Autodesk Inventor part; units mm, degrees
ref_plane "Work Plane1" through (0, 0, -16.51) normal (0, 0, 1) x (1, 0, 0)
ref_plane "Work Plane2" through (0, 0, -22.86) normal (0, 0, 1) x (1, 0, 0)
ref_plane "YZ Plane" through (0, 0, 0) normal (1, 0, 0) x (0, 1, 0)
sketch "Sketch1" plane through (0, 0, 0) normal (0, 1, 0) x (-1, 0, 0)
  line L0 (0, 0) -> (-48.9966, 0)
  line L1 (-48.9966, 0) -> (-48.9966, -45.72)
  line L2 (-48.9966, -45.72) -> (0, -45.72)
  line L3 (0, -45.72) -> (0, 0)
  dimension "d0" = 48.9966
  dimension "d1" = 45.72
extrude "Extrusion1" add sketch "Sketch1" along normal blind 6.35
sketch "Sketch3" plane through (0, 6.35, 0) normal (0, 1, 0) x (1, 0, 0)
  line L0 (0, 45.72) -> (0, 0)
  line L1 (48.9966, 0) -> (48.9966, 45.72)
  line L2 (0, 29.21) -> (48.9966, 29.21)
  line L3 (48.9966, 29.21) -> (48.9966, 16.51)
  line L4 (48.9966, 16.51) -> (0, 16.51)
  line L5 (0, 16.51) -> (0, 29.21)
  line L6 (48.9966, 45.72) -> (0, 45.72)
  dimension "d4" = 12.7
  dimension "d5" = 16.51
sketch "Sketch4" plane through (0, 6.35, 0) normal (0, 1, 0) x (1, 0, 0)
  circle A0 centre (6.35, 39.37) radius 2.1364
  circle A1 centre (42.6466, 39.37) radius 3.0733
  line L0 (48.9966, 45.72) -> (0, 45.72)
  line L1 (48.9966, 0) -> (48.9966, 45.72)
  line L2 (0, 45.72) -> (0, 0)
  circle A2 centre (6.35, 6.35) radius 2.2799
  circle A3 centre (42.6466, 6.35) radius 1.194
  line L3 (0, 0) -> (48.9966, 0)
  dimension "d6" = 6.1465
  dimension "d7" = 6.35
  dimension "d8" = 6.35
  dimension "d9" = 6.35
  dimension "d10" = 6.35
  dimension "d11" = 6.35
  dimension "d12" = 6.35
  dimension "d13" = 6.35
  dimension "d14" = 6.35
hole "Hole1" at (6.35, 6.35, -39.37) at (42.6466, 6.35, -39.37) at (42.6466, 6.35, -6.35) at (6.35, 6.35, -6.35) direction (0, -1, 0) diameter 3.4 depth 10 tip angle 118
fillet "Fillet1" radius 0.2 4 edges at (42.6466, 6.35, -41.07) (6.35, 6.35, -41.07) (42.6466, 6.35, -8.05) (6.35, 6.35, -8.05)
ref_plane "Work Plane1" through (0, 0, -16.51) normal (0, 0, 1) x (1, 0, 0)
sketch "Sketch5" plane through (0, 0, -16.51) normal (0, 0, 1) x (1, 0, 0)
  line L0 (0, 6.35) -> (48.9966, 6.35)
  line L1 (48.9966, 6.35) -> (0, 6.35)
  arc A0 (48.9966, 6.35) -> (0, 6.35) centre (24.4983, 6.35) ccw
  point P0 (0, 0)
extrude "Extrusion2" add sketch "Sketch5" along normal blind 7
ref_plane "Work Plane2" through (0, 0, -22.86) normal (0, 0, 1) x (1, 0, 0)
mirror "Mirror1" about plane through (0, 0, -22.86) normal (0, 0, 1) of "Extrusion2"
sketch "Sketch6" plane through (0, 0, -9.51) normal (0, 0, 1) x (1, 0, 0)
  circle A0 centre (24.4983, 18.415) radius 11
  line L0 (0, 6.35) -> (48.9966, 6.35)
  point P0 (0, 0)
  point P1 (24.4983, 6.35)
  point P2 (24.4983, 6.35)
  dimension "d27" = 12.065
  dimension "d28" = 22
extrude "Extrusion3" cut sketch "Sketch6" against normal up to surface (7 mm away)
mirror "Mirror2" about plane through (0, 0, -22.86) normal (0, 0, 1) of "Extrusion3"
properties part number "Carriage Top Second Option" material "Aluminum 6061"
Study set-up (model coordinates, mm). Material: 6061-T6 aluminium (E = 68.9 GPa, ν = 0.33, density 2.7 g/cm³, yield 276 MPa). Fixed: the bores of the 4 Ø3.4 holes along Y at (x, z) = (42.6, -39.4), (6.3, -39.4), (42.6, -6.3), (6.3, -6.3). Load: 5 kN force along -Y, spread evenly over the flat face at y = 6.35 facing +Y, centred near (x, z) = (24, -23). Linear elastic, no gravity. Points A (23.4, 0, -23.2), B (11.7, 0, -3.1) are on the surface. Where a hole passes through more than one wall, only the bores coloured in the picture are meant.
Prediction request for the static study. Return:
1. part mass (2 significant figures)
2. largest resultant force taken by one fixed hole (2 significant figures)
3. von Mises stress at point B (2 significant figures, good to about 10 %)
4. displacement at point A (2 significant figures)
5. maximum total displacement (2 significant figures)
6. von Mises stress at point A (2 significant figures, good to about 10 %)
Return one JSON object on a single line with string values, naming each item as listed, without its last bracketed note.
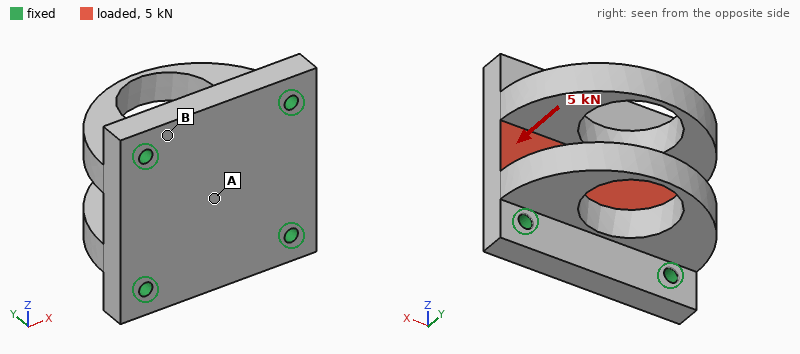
{"part mass": "59 g", "largest resultant force taken by one fixed hole": "1.3 kN", "von Mises stress at point B": "19 MPa", "displacement at point A": "26 µm", "maximum total displacement": "44 µm", "von Mises stress at point A": "46 MPa"}
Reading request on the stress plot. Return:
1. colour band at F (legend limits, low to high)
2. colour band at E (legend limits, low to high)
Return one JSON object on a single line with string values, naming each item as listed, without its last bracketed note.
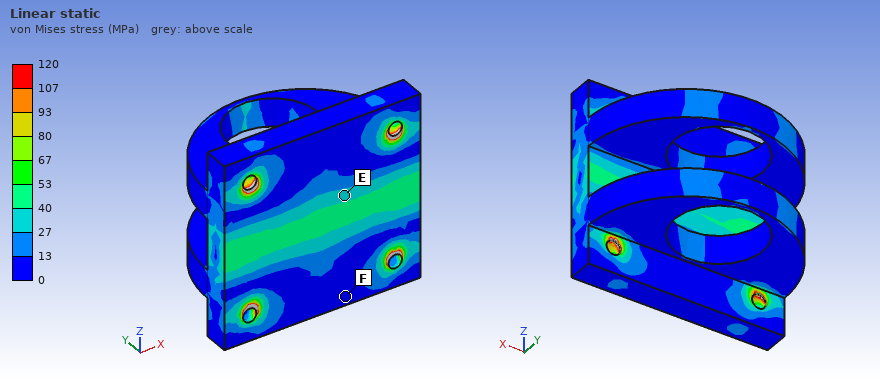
{"colour band at F": "0 to 13 MPa", "colour band at E": "27 to 40 MPa"}
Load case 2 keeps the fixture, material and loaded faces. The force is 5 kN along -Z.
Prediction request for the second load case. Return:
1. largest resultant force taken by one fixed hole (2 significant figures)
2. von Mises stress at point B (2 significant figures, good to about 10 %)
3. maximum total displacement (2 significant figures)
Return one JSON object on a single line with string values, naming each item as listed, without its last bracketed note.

{"largest resultant force taken by one fixed hole": "1.3 kN", "von Mises stress at point B": "7.0 MPa", "maximum total displacement": "5.0 µm"}
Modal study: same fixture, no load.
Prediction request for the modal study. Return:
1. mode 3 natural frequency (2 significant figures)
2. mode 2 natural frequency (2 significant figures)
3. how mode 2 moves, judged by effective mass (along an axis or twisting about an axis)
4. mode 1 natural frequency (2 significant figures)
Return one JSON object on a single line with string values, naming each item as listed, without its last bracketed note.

{"mode 3 natural frequency": "13 kHz", "mode 2 natural frequency": "10 kHz", "how mode 2 moves, judged by effective mass": "along Z", "mode 1 natural frequency": "8300 Hz"}
